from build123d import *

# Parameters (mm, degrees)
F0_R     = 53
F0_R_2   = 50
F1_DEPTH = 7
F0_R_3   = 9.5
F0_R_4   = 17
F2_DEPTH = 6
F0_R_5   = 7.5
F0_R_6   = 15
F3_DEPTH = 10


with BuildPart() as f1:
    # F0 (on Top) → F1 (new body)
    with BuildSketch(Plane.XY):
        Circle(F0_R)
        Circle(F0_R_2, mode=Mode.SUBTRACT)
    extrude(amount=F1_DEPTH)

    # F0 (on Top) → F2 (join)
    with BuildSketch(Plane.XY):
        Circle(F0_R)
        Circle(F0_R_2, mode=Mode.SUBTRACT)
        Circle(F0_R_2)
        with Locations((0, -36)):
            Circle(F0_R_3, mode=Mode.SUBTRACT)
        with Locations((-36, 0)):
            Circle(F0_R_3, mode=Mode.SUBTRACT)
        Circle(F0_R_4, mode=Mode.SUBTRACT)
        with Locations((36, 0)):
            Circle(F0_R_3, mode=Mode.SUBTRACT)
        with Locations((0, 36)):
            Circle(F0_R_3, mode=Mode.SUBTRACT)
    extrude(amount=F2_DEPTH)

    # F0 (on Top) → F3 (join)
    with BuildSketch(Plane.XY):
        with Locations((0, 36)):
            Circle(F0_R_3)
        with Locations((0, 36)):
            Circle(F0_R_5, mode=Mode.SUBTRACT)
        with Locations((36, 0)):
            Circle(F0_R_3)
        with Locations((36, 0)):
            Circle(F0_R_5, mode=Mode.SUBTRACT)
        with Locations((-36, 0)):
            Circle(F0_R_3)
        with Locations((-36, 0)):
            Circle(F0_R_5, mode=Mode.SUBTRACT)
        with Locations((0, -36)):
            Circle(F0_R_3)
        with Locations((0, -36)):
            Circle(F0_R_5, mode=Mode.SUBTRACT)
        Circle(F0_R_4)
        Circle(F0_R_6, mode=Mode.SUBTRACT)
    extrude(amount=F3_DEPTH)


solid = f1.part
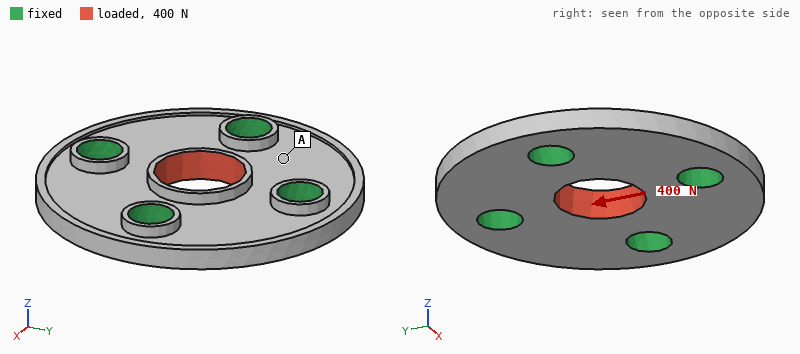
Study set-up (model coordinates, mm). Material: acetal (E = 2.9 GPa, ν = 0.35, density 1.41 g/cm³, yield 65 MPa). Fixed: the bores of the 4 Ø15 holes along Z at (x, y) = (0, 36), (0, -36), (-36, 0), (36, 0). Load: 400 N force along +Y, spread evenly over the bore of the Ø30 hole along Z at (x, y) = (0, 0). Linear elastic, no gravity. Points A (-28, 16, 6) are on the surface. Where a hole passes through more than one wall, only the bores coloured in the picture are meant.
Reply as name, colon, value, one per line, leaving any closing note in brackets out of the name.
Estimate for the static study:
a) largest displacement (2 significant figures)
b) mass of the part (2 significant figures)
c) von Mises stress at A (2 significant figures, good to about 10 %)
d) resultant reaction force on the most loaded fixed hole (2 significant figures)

largest displacement: 15 µm
mass of the part: 68 g
von Mises stress at A: 0.26 MPa
resultant reaction force on the most loaded fixed hole: 130 N
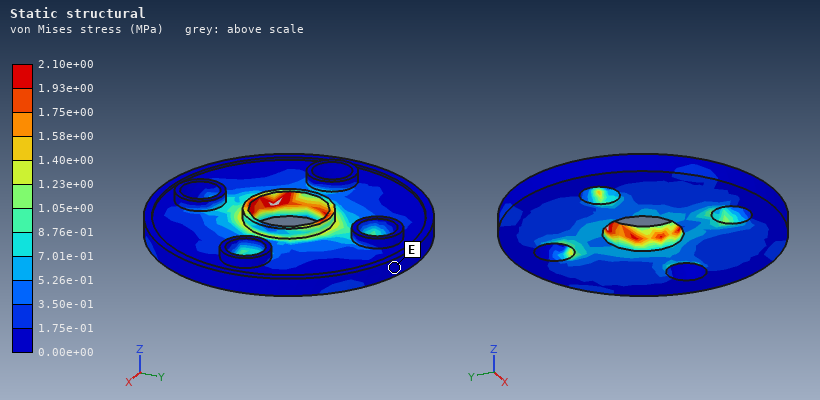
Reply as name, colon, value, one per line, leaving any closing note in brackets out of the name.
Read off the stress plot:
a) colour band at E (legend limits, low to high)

colour band at E: 0.00e+00 to 1.75e-01 MPa
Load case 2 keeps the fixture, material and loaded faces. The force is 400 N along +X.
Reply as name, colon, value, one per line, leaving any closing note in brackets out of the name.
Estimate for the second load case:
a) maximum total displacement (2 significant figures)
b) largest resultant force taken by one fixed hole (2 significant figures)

maximum total displacement: 15 µm
largest resultant force taken by one fixed hole: 130 N
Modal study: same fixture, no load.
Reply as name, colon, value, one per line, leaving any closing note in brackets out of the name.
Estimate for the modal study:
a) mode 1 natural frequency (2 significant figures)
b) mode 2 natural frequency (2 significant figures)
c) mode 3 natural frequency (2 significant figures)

mode 1 natural frequency: 2600 Hz
mode 2 natural frequency: 2700 Hz
mode 3 natural frequency: 2700 Hz
